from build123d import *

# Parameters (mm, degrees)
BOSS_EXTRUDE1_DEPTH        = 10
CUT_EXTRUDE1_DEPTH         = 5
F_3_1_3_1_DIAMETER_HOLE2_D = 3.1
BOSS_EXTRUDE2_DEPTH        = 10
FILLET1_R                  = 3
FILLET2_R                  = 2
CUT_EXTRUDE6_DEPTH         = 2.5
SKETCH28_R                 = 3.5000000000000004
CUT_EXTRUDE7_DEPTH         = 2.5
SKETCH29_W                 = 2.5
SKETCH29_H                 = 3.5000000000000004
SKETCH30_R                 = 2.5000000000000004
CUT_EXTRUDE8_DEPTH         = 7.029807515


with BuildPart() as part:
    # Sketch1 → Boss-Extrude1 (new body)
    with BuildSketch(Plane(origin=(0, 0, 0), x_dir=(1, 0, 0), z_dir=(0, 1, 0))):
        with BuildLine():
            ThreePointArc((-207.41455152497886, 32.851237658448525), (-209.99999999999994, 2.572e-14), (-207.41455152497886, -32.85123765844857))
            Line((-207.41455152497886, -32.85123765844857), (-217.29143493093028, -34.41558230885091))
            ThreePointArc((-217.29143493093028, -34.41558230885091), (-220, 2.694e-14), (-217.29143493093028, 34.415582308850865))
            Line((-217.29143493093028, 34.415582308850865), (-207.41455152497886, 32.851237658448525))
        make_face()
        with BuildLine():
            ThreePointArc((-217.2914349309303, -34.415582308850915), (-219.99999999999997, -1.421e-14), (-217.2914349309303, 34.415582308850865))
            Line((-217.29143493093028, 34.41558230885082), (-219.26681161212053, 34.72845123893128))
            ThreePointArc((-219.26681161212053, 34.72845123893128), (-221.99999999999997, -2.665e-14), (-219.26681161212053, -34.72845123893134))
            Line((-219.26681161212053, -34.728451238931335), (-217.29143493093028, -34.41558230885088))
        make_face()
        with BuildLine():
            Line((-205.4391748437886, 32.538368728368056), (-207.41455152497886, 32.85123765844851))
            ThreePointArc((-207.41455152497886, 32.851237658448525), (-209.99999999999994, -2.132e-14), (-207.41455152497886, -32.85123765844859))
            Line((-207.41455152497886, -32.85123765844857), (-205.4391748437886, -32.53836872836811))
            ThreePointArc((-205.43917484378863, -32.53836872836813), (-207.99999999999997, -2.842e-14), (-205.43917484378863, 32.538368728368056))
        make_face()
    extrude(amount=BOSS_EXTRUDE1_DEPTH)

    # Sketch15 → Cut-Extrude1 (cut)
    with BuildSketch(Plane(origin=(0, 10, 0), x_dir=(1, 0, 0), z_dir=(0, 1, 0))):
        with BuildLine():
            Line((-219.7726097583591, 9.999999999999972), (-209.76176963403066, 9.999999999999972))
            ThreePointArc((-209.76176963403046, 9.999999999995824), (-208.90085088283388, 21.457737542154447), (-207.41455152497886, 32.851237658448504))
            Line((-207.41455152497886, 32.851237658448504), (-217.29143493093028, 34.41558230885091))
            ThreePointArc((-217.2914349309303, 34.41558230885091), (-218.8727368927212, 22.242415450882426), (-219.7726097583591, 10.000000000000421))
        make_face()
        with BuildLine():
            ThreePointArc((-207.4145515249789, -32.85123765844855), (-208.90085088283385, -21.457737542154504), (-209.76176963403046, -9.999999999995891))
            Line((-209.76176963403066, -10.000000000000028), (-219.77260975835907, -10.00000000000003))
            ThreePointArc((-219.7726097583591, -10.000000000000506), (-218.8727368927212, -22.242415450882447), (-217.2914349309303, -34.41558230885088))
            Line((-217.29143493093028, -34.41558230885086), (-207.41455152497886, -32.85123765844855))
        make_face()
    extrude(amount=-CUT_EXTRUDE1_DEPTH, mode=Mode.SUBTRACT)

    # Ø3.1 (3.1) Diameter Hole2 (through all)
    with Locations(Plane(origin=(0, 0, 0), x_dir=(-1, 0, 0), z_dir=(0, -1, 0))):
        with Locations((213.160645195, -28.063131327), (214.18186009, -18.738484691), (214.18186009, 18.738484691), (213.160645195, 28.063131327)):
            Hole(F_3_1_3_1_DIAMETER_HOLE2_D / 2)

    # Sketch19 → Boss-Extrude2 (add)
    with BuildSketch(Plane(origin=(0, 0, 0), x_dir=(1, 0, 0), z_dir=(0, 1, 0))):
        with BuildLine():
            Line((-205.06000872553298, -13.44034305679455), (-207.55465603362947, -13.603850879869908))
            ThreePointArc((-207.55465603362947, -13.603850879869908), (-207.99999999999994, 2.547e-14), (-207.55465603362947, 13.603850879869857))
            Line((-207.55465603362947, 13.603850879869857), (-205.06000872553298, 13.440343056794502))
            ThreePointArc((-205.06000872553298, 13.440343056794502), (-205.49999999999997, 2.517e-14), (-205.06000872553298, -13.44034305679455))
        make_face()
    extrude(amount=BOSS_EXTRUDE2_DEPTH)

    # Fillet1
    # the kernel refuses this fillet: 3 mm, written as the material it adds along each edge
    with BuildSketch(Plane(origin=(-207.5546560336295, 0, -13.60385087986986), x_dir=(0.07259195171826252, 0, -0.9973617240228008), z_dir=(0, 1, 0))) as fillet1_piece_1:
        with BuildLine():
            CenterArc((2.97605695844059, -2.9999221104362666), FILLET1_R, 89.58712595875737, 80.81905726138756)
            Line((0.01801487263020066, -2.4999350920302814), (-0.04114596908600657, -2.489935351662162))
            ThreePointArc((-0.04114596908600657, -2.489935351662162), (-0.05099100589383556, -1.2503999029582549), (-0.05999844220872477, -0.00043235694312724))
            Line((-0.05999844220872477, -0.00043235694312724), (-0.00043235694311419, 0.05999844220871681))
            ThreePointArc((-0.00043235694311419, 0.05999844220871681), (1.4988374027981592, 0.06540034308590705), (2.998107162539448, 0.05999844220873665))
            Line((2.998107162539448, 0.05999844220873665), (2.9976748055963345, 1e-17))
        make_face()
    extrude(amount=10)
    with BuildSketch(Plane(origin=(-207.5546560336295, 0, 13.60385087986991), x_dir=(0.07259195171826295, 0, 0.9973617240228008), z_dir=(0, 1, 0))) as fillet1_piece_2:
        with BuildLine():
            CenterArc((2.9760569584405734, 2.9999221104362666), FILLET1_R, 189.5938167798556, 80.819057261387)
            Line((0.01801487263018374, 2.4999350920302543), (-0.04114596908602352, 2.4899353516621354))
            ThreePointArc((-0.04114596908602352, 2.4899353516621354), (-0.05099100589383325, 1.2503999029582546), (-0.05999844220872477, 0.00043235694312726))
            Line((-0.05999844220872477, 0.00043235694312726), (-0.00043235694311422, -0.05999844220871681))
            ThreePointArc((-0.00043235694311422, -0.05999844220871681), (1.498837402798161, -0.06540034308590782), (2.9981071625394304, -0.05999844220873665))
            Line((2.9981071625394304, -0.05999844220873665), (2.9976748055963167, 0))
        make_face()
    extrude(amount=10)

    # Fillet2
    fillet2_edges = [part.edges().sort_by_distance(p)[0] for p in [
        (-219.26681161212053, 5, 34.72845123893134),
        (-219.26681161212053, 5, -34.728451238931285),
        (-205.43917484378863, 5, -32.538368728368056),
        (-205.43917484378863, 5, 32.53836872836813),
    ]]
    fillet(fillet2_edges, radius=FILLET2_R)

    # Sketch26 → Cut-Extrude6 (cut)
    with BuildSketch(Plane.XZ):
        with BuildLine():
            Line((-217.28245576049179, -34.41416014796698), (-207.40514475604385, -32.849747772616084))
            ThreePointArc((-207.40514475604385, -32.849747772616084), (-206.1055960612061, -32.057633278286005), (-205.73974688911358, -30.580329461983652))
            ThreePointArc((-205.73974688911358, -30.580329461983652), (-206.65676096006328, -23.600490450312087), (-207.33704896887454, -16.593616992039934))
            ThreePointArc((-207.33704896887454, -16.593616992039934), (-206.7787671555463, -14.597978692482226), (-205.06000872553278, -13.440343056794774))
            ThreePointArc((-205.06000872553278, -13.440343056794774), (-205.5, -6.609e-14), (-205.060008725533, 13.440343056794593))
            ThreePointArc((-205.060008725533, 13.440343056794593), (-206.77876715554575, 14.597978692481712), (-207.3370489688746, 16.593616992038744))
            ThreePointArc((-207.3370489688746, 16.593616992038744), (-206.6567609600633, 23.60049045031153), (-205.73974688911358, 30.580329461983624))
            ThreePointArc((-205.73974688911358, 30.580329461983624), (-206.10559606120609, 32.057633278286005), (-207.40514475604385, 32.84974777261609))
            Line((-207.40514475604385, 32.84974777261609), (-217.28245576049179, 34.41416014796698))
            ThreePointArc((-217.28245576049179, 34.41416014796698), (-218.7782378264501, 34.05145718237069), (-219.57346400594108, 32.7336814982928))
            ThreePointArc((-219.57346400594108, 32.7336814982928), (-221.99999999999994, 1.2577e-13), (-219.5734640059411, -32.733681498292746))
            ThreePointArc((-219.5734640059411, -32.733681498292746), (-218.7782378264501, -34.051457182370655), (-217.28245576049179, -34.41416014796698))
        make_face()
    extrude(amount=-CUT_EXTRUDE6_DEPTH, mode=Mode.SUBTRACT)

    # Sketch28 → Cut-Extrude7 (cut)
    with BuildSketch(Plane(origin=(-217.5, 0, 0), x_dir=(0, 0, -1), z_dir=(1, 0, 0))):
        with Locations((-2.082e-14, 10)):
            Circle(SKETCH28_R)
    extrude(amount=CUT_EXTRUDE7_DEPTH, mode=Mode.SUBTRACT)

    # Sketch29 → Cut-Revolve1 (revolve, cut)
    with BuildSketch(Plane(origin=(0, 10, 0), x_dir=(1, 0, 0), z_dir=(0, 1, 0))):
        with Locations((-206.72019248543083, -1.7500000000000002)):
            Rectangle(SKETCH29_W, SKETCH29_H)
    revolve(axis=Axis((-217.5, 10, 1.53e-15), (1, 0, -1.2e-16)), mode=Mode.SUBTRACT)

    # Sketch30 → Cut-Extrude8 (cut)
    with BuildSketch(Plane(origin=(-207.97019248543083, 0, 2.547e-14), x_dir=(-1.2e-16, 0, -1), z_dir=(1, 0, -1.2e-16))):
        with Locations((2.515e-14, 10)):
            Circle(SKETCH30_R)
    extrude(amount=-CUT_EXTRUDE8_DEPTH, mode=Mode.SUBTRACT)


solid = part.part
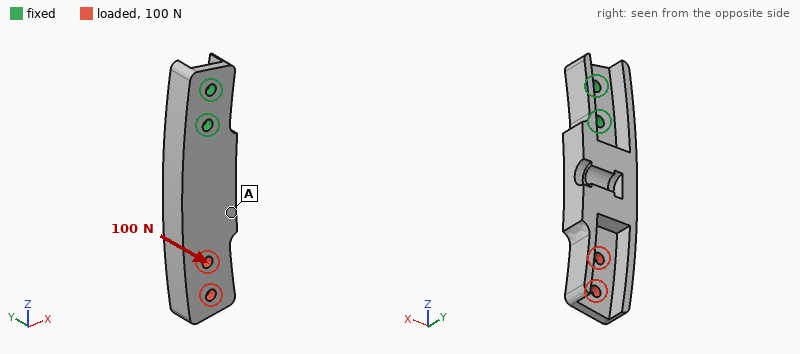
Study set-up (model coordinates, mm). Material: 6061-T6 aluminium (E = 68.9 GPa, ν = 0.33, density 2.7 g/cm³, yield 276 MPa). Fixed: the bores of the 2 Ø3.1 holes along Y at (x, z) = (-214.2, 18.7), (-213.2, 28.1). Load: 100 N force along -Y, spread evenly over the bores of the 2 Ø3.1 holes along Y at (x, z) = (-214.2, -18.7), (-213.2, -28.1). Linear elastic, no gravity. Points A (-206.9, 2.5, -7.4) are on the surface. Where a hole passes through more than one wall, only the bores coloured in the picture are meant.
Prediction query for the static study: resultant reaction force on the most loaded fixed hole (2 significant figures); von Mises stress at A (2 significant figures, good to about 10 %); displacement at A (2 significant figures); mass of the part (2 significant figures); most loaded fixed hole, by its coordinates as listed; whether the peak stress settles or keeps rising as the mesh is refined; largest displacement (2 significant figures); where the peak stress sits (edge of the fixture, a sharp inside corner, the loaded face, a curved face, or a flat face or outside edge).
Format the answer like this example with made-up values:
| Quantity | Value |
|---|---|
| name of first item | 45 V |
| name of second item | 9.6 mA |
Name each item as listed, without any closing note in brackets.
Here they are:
| Quantity | Value |
|---|---|
| resultant reaction force on the most loaded fixed hole | 430 N |
| von Mises stress at A | 10 MPa |
| displacement at A | 0.11 mm |
| mass of the part | 13 g |
| most loaded fixed hole, by its coordinates as listed | (-214.2, 18.7) |
| whether the peak stress settles or keeps rising as the mesh is refined | keeps rising |
| largest displacement | 0.26 mm |
| where the peak stress sits | edge of the fixture |
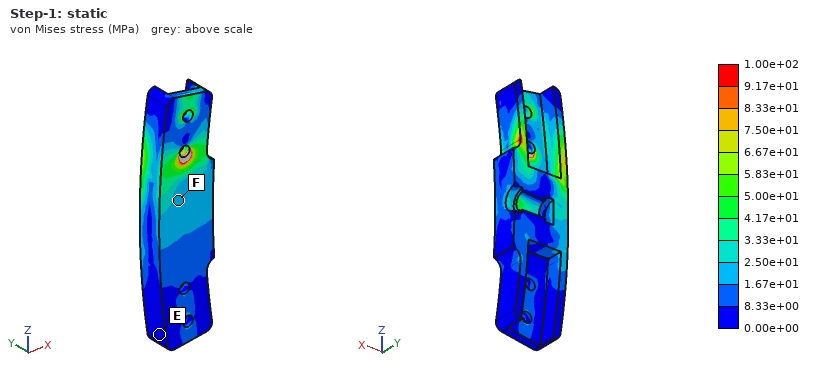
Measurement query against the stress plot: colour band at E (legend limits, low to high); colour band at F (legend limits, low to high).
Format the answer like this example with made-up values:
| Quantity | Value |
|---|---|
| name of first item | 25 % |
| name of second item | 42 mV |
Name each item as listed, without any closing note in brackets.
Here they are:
| Quantity | Value |
|---|---|
| colour band at E | 0.00e+00 to 8.33e+00 MPa |
| colour band at F | 1.67e+01 to 2.50e+01 MPa |
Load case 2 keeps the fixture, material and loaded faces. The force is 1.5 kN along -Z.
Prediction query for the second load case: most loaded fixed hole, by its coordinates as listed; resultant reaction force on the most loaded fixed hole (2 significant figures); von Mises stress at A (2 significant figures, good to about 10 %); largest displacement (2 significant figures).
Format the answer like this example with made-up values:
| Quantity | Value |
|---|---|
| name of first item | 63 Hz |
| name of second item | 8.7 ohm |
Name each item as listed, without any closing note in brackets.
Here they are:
| Quantity | Value |
|---|---|
| most loaded fixed hole, by its coordinates as listed | (-214.2, 18.7) |
| resultant reaction force on the most loaded fixed hole | 1.2 kN |
| von Mises stress at A | 35 MPa |
| largest displacement | 0.14 mm |
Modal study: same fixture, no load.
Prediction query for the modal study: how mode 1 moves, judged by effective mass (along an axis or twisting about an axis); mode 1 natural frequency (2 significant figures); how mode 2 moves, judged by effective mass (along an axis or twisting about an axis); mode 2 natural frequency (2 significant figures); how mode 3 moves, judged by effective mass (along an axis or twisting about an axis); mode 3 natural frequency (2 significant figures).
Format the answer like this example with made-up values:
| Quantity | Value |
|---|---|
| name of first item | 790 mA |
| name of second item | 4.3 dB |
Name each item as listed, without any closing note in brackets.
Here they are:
| Quantity | Value |
|---|---|
| how mode 1 moves, judged by effective mass | along Y |
| mode 1 natural frequency | 1700 Hz |
| how mode 2 moves, judged by effective mass | along X |
| mode 2 natural frequency | 3400 Hz |
| how mode 3 moves, judged by effective mass | twisting about Z |
| mode 3 natural frequency | 5800 Hz |
